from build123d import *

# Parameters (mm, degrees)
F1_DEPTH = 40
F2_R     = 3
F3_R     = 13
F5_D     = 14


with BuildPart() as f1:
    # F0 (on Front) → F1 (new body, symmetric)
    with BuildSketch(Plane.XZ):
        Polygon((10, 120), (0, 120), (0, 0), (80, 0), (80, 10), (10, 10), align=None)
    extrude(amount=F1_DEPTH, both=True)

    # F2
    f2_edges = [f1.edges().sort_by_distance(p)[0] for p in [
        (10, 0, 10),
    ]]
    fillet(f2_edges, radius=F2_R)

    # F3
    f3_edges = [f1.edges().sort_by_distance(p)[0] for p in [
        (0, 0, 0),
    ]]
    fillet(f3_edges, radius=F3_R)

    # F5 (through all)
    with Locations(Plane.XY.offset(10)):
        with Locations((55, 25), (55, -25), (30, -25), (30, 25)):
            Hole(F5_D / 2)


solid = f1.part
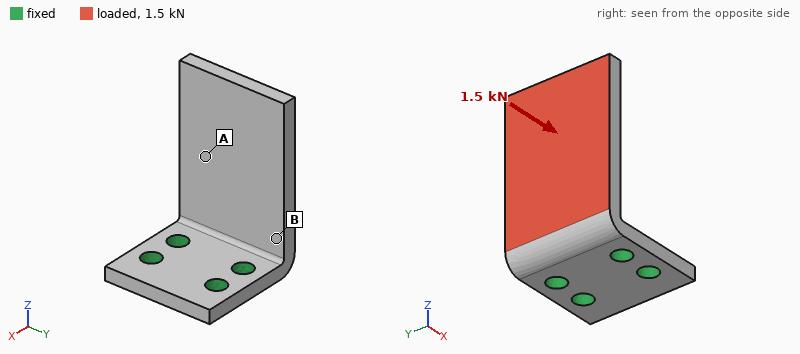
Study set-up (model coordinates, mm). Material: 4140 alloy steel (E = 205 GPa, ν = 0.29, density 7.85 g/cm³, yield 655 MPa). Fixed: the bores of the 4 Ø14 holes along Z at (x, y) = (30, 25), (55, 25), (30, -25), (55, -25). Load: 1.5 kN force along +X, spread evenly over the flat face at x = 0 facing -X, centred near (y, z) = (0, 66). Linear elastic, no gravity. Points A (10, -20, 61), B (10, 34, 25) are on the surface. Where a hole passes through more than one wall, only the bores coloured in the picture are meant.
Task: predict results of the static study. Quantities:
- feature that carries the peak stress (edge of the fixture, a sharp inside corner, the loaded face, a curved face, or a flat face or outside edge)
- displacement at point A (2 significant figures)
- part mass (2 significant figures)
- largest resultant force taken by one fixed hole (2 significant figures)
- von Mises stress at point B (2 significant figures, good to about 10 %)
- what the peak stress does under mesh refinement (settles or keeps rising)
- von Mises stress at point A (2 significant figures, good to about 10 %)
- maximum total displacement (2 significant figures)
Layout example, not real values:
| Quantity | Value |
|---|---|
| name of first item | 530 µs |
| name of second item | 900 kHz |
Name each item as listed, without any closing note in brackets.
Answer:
| Quantity | Value |
|---|---|
| feature that carries the peak stress | edge of the fixture |
| displacement at point A | 0.14 mm |
| part mass | 1.1 kg |
| largest resultant force taken by one fixed hole | 710 N |
| von Mises stress at point B | 44 MPa |
| what the peak stress does under mesh refinement | keeps rising |
| von Mises stress at point A | 18 MPa |
| maximum total displacement | 0.35 mm |
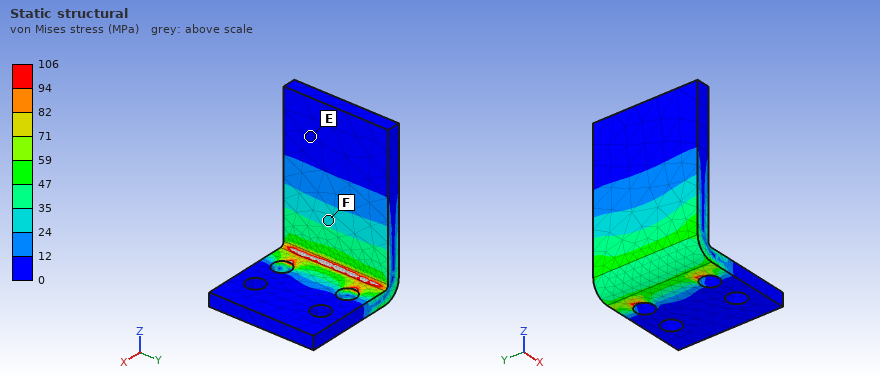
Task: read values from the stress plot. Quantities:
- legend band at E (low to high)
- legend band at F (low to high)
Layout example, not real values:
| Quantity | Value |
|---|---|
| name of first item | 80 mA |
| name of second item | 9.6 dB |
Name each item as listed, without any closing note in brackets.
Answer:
| Quantity | Value |
|---|---|
| legend band at E | 0 to 12 MPa |
| legend band at F | 24 to 35 MPa |
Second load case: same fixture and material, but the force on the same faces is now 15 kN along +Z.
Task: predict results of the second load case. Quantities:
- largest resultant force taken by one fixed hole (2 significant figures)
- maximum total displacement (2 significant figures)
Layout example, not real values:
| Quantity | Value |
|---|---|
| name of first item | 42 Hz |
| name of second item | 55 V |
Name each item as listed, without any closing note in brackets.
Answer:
| Quantity | Value |
|---|---|
| largest resultant force taken by one fixed hole | 8.6 kN |
| maximum total displacement | 0.67 mm |
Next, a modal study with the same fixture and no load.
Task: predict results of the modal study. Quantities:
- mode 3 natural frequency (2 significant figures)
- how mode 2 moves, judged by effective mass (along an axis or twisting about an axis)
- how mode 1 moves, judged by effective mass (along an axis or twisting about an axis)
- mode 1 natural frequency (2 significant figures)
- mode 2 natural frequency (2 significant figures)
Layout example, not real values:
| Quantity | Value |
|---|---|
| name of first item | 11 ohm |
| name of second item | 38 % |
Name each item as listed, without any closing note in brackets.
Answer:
| Quantity | Value |
|---|---|
| mode 3 natural frequency | 2100 Hz |
| how mode 2 moves, judged by effective mass | along Y |
| how mode 1 moves, judged by effective mass | along X |
| mode 1 natural frequency | 500 Hz |
| mode 2 natural frequency | 1500 Hz |
